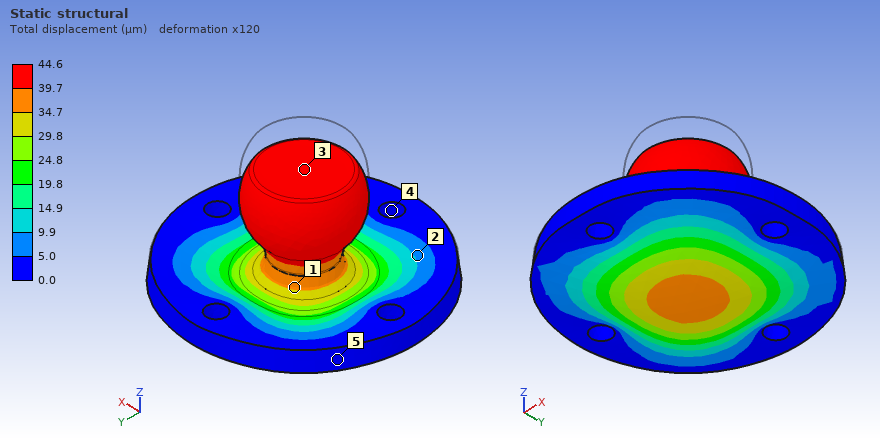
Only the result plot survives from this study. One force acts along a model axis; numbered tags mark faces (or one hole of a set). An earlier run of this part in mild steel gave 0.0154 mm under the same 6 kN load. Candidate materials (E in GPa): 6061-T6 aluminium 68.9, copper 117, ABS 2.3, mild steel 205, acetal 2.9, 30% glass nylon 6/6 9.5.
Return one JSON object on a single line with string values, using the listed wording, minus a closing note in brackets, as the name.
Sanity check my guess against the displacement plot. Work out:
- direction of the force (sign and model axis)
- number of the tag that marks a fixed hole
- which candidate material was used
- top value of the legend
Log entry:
{"direction of the force": "-Z", "number of the tag that marks a fixed hole": "4", "which candidate material was used": "6061-T6 aluminium", "top value of the legend": "44.6 µm"}
